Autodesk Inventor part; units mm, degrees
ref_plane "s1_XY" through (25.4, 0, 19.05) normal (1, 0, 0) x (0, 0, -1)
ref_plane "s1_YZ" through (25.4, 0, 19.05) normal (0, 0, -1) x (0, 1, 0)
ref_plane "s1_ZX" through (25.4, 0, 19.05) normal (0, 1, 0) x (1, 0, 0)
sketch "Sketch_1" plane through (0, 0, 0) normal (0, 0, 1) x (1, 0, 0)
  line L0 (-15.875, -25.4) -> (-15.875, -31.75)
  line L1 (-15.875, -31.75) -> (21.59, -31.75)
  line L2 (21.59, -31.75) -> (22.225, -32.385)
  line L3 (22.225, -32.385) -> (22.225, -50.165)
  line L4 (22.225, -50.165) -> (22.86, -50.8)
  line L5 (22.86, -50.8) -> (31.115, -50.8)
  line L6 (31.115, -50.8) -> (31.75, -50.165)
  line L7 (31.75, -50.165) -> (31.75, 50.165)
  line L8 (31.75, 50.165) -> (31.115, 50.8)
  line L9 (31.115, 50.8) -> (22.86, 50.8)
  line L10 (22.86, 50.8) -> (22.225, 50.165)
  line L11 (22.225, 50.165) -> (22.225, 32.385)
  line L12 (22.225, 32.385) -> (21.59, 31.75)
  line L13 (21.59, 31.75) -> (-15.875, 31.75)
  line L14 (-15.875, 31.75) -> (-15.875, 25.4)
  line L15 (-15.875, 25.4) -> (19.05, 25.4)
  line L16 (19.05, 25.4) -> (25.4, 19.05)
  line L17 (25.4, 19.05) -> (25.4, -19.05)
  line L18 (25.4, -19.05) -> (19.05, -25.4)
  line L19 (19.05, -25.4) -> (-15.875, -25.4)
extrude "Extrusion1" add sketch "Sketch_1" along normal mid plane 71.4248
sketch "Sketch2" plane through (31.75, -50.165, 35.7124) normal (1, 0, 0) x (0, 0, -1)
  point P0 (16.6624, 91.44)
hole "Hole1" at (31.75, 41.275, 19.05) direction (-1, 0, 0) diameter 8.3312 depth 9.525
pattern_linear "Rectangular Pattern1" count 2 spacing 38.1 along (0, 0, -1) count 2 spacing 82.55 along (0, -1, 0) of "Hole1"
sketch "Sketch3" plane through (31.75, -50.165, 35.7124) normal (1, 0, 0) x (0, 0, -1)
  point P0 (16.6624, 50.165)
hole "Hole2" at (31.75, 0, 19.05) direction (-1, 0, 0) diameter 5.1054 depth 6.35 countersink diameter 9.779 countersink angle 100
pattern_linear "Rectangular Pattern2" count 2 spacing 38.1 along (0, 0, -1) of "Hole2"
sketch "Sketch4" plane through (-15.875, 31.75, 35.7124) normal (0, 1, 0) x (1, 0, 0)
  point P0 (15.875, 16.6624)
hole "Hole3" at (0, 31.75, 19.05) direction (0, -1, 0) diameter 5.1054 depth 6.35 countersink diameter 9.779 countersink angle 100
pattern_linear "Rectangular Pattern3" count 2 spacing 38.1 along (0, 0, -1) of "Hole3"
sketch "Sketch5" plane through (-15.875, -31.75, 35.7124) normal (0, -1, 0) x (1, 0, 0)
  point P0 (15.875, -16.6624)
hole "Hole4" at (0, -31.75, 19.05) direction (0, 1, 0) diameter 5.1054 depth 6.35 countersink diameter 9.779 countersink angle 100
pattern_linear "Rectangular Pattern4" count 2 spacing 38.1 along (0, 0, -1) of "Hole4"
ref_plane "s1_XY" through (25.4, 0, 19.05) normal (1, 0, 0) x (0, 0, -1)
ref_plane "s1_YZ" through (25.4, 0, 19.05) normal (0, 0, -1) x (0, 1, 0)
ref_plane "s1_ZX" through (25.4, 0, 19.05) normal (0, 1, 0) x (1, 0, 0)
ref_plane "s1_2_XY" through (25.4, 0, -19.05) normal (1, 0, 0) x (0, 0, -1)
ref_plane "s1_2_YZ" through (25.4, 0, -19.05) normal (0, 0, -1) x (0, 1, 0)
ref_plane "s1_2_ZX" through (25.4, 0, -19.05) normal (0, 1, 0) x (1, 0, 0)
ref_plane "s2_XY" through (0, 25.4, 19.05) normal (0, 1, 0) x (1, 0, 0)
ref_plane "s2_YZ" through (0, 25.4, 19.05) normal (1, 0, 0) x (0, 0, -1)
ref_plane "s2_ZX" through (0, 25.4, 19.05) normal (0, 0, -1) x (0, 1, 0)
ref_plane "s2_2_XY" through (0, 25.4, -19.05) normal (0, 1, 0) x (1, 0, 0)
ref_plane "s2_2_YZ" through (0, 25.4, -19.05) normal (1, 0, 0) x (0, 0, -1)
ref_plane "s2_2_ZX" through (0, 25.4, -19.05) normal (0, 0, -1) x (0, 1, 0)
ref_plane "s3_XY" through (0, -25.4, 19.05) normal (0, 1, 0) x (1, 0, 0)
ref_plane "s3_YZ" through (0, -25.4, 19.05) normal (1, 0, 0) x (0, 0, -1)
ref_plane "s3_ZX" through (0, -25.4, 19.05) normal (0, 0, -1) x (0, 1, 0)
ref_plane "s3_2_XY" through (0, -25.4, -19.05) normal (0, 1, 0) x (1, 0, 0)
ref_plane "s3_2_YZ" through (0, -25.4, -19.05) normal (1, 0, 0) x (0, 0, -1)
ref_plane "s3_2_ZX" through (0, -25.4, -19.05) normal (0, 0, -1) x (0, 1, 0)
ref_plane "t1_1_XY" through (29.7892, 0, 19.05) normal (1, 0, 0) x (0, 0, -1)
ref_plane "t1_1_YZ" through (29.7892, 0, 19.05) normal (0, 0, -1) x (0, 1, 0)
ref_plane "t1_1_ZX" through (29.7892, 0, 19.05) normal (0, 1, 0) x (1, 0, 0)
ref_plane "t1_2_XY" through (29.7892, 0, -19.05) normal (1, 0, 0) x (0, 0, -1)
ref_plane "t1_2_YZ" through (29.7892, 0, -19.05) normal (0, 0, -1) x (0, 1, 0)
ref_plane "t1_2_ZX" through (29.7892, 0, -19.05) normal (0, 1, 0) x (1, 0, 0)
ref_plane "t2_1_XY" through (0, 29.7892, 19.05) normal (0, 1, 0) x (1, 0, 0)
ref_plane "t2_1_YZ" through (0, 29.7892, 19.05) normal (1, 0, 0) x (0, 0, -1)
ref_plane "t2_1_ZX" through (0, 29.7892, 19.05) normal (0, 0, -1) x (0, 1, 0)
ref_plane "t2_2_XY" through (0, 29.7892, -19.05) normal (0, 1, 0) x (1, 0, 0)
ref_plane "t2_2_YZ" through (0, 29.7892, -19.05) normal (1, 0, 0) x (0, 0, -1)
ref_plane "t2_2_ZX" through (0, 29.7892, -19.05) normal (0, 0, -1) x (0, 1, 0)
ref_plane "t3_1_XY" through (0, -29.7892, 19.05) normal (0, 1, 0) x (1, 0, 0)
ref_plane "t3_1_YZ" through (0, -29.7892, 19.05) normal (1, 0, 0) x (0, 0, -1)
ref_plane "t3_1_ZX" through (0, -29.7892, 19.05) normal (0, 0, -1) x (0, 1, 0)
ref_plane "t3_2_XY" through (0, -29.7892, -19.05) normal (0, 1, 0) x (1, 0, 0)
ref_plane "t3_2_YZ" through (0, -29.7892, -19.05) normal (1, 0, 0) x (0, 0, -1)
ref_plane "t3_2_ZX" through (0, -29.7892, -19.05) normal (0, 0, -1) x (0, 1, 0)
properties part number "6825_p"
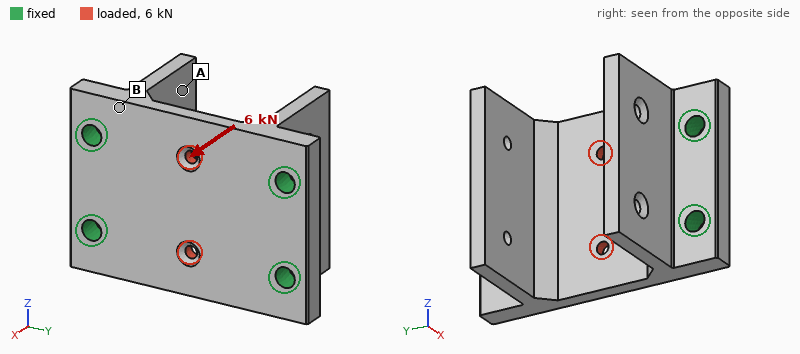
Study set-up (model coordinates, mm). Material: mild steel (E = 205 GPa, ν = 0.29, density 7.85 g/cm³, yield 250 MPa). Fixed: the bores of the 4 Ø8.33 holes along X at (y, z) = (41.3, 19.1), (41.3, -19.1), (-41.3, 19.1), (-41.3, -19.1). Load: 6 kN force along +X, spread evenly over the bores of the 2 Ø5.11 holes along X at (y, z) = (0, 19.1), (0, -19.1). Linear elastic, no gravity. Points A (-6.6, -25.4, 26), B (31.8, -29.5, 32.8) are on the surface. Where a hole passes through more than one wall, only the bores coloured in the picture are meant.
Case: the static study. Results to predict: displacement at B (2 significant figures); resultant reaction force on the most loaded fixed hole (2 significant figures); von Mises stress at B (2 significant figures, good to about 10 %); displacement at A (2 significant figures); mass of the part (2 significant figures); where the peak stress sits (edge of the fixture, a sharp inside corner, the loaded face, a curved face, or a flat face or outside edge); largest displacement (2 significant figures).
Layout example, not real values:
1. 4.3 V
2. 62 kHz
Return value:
1. 5.7 µm
2. 2.1 kN
3. 24 MPa
4. 26 µm
5. 720 g
6. the loaded face
7. 35 µm
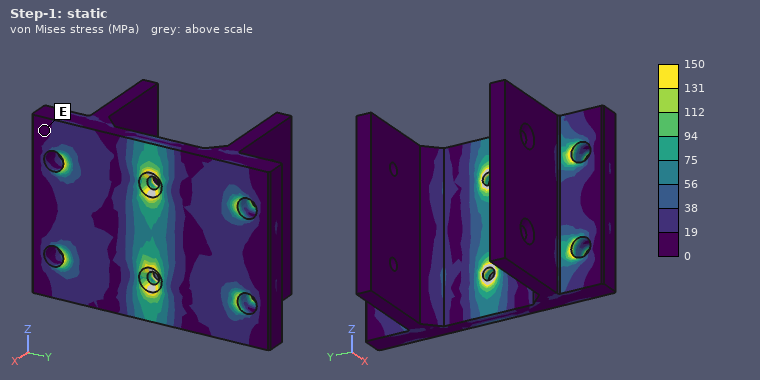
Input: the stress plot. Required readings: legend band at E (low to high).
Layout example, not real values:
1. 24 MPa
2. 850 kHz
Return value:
1. 0 to 19 MPa
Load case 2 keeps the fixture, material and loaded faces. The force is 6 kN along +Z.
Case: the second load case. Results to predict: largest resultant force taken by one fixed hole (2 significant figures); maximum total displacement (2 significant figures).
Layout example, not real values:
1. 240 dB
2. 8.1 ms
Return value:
1. 1.8 kN
2. 4.8 µm
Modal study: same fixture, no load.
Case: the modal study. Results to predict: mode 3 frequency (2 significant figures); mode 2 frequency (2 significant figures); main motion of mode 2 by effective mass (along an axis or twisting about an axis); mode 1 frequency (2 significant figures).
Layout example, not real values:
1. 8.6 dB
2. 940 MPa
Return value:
1. 4800 Hz
2. 3300 Hz
3. along Y
4. 2900 Hz
